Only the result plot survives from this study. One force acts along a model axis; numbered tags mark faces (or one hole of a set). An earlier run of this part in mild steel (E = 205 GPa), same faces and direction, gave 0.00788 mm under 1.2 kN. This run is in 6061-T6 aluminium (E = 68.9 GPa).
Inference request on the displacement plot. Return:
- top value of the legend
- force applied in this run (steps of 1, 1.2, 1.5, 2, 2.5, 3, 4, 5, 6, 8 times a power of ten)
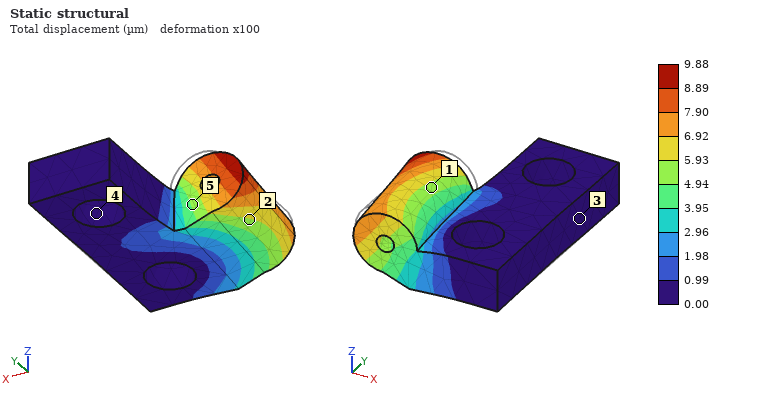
9.88 µm
500 N
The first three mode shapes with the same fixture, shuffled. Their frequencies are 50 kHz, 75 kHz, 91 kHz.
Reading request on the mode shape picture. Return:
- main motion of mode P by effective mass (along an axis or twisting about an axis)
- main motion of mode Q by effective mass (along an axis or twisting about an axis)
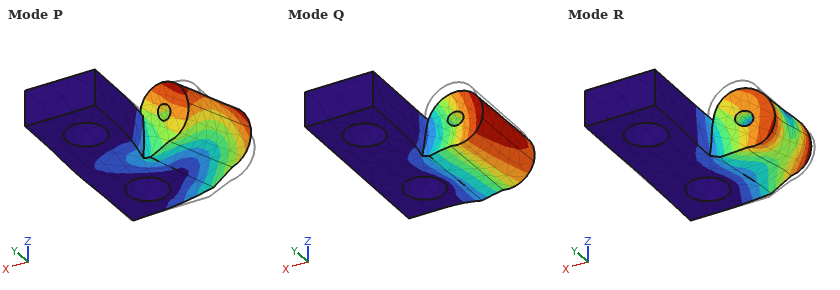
along Y
along Z
